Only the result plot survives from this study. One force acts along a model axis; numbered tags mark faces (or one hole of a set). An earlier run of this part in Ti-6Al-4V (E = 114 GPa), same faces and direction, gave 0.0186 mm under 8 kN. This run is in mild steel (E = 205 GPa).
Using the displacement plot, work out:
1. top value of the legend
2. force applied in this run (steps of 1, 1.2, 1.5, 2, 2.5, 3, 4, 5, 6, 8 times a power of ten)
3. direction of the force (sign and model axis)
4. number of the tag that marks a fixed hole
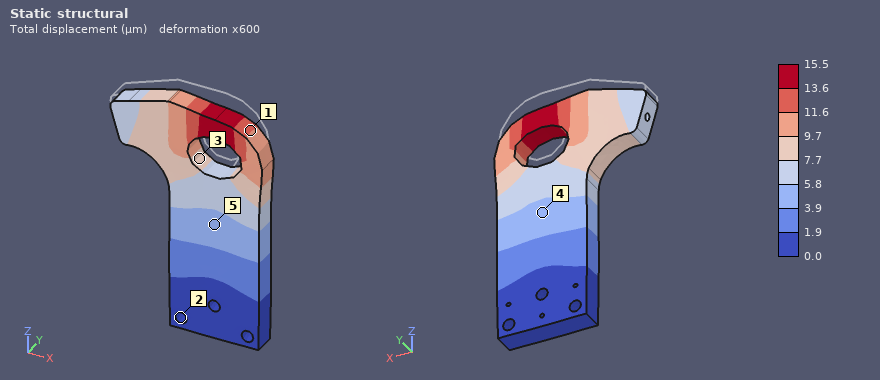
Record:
15.5 µm
12 kN
-Z
2
